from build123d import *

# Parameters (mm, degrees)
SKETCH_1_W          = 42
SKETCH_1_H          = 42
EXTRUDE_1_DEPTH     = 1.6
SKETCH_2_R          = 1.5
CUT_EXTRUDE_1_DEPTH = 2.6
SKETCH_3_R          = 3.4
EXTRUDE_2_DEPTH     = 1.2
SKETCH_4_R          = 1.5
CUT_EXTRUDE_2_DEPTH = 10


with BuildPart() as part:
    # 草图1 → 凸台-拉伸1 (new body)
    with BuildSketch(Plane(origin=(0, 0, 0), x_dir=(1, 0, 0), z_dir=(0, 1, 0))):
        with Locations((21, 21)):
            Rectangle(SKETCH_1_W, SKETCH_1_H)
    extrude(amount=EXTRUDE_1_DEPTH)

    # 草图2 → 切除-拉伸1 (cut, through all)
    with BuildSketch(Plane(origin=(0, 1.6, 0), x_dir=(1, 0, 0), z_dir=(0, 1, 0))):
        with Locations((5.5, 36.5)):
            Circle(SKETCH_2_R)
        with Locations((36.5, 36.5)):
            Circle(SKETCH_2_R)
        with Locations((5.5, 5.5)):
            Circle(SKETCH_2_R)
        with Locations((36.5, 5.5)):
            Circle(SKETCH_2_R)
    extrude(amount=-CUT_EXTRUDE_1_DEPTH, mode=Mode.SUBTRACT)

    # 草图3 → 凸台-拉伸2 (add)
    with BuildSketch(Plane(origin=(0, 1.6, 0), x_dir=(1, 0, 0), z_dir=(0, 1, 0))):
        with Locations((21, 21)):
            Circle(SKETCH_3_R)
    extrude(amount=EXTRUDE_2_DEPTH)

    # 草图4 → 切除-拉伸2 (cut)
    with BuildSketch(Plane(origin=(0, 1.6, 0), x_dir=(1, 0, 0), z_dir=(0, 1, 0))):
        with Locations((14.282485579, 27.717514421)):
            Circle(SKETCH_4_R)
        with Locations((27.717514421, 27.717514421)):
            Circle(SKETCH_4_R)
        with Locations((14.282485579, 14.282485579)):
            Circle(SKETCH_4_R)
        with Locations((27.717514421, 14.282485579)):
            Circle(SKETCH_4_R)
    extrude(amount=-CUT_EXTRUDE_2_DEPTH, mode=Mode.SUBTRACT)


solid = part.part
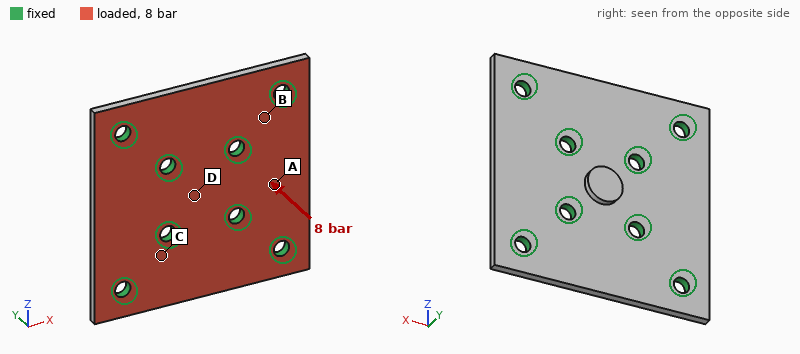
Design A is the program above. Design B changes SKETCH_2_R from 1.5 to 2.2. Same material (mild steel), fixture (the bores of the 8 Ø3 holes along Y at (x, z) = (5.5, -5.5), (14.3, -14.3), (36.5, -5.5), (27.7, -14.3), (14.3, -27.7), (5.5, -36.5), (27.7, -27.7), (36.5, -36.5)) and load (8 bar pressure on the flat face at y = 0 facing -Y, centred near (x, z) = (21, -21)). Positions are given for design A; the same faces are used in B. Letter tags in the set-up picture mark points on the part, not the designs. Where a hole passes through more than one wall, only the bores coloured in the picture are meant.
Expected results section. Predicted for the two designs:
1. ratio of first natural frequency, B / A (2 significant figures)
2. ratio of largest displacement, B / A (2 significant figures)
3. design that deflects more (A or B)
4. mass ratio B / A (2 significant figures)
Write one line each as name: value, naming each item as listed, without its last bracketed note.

ratio of first natural frequency, B / A: 1.1
ratio of largest displacement, B / A: 0.89
design that deflects more: A
mass ratio B / A: 0.98
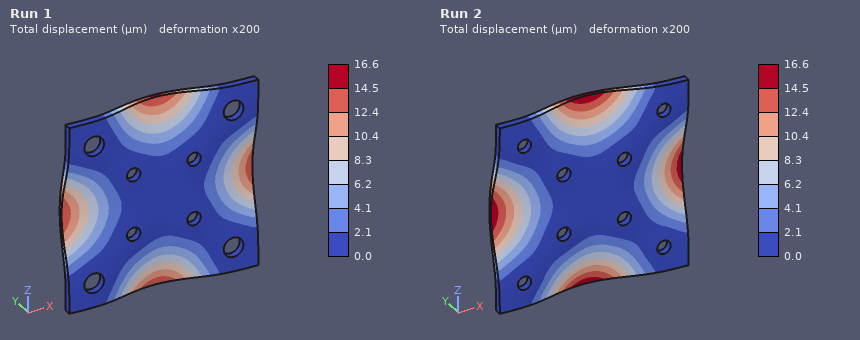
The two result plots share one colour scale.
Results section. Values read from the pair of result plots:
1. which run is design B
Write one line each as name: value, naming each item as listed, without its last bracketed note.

which run is design B: Run 1
